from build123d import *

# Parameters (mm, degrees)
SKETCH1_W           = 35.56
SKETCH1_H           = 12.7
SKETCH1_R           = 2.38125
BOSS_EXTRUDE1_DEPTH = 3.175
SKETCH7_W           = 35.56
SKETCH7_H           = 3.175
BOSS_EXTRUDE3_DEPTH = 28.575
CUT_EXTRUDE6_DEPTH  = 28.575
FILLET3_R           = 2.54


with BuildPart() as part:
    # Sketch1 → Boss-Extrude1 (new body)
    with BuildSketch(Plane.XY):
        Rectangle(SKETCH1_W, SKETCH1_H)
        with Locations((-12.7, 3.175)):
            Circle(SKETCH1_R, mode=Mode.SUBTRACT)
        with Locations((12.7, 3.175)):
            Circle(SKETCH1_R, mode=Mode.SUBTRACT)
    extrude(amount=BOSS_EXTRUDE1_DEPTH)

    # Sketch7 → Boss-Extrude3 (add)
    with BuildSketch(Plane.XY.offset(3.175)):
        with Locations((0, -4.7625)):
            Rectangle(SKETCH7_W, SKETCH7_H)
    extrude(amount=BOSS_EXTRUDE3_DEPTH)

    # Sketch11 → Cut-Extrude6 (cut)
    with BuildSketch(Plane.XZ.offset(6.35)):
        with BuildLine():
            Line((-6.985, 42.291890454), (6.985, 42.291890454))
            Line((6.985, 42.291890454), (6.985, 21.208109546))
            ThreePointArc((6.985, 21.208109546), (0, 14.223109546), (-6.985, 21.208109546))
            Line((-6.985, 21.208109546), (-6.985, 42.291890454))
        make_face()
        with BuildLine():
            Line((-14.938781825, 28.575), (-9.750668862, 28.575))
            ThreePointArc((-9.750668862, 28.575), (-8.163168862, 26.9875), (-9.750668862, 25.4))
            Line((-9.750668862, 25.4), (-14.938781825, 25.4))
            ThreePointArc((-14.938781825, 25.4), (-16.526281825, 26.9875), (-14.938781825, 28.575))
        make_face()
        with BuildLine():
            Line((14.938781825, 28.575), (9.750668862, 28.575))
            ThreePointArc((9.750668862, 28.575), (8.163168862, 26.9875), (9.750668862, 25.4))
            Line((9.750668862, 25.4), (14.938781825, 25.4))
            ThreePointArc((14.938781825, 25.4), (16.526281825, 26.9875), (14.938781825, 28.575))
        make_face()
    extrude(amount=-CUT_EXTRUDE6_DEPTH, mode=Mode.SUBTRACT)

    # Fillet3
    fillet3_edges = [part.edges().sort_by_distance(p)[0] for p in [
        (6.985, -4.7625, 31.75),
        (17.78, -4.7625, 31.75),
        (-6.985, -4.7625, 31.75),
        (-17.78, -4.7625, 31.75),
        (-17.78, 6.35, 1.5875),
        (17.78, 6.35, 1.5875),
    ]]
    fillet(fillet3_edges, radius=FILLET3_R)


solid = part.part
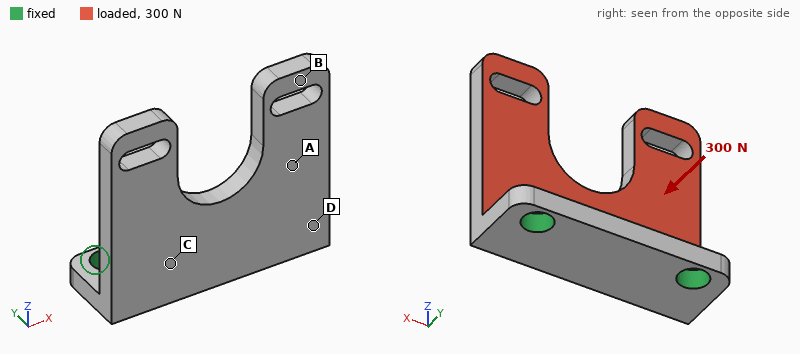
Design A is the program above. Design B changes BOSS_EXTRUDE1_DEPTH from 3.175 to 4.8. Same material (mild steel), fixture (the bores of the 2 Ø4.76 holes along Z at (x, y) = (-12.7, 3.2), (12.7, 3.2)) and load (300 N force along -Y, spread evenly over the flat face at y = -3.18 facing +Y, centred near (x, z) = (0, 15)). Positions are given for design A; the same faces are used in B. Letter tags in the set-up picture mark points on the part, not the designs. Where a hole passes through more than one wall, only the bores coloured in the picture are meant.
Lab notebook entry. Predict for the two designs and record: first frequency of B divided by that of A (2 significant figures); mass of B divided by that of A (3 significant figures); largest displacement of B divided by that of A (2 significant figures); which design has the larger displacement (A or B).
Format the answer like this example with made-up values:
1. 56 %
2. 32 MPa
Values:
1. 1.3
2. 1.13
3. 0.61
4. A
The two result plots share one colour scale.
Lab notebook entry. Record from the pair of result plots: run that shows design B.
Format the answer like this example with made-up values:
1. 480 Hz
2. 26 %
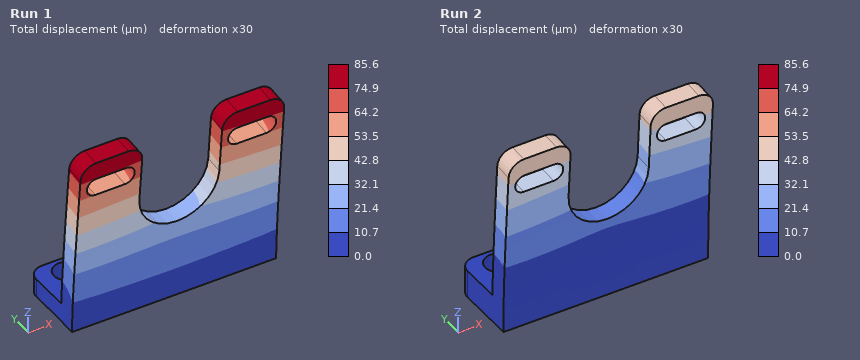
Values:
1. Run 2
